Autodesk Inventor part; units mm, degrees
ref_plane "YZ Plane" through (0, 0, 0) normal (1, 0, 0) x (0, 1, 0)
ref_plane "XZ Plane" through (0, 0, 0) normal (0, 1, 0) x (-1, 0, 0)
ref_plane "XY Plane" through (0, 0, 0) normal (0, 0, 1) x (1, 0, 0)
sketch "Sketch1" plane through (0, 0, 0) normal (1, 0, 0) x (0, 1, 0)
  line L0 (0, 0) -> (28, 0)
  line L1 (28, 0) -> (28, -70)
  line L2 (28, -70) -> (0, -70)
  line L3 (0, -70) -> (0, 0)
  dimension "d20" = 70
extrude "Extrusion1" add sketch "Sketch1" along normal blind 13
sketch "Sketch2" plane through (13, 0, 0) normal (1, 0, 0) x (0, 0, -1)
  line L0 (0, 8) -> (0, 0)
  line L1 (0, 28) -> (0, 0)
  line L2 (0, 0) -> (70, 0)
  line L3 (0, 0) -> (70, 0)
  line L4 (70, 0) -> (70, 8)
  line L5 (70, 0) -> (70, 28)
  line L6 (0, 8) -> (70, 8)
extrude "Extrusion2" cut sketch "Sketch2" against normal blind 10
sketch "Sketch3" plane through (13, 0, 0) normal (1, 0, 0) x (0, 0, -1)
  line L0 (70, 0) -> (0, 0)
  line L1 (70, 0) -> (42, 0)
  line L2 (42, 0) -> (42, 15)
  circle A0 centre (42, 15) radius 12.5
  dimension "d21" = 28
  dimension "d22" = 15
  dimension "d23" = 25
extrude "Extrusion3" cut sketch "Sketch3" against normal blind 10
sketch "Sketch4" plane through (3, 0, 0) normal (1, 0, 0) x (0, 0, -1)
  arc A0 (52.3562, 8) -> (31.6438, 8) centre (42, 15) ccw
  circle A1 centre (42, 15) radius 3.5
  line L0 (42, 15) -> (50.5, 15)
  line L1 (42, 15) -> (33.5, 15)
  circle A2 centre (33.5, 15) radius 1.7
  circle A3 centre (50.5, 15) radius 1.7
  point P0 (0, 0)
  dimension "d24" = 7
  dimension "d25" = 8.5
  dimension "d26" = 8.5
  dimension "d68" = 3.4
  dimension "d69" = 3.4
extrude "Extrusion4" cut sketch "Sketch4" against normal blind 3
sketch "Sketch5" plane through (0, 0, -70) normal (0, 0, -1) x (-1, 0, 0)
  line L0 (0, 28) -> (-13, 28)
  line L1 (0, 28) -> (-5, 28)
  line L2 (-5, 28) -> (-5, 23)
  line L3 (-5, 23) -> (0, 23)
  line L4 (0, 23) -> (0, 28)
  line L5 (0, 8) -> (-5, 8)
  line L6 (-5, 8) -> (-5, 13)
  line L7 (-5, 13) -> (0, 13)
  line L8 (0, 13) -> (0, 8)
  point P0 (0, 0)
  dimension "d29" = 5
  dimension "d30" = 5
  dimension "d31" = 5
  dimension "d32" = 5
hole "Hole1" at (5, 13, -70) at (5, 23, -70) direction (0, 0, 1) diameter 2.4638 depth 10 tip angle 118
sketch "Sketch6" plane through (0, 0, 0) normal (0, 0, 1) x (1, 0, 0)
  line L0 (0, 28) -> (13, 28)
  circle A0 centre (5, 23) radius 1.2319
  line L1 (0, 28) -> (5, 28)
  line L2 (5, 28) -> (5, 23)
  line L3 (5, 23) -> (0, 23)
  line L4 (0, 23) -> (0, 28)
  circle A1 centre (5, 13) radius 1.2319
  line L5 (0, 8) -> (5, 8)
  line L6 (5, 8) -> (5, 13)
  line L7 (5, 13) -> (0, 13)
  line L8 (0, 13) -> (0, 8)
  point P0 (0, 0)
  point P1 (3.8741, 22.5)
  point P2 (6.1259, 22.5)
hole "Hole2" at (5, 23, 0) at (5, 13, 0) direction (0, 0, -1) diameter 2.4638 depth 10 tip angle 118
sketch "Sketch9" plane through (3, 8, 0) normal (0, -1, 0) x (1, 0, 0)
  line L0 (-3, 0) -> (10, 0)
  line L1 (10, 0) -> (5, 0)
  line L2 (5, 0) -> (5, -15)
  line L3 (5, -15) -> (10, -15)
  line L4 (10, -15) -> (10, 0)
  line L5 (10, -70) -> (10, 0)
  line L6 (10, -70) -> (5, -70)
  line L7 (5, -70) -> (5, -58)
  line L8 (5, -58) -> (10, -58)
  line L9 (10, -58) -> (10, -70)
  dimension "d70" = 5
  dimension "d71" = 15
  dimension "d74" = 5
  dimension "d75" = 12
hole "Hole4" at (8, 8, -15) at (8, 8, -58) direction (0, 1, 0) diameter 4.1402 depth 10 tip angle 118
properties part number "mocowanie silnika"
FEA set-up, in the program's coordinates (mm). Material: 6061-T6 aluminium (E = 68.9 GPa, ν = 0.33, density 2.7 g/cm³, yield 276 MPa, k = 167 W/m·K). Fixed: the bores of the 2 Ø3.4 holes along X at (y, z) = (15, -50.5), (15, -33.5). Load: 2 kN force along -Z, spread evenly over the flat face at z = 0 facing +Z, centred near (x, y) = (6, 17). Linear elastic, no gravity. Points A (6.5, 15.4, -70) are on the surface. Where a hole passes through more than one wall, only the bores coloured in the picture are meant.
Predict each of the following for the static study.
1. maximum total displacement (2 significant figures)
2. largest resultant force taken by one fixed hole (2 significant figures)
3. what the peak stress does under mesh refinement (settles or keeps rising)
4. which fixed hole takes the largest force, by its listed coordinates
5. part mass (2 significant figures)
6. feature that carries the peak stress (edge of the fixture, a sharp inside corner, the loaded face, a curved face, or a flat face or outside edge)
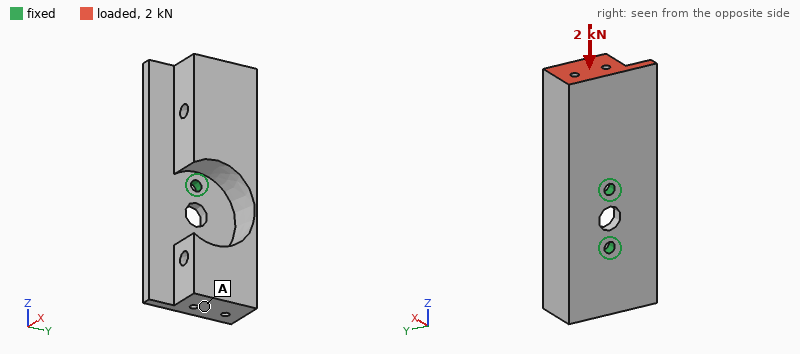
0.17 mm
1.4 kN
keeps rising
(15, -33.5)
41 g
edge of the fixture
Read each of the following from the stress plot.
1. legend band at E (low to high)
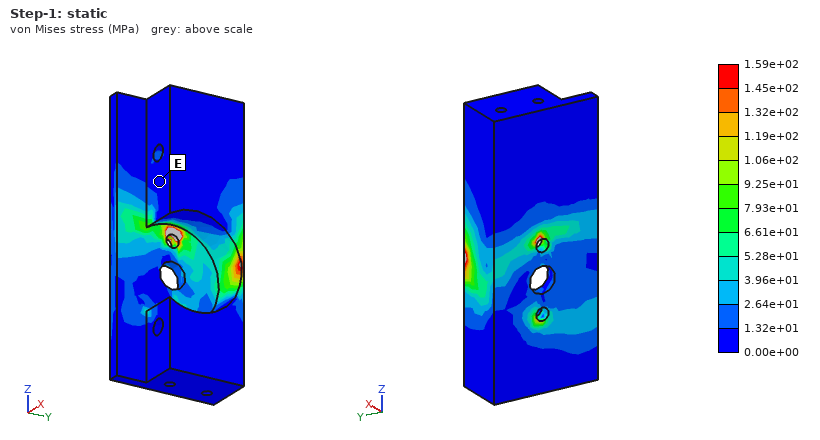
0.00e+00 to 1.32e+01 MPa
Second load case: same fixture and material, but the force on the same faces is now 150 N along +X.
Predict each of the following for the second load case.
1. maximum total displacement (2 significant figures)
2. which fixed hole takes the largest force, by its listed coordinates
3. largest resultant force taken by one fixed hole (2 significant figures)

98 µm
(15, -33.5)
320 N
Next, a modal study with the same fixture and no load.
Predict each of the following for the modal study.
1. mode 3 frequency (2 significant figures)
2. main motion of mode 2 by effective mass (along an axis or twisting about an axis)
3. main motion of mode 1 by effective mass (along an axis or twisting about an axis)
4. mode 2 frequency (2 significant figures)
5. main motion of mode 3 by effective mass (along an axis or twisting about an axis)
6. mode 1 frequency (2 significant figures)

5000 Hz
along Y
along X
4300 Hz
along X
2200 Hz
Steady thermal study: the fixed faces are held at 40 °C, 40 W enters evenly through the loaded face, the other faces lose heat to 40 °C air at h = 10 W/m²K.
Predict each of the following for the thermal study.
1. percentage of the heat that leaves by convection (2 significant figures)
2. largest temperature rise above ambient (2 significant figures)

3.1 %
48 K
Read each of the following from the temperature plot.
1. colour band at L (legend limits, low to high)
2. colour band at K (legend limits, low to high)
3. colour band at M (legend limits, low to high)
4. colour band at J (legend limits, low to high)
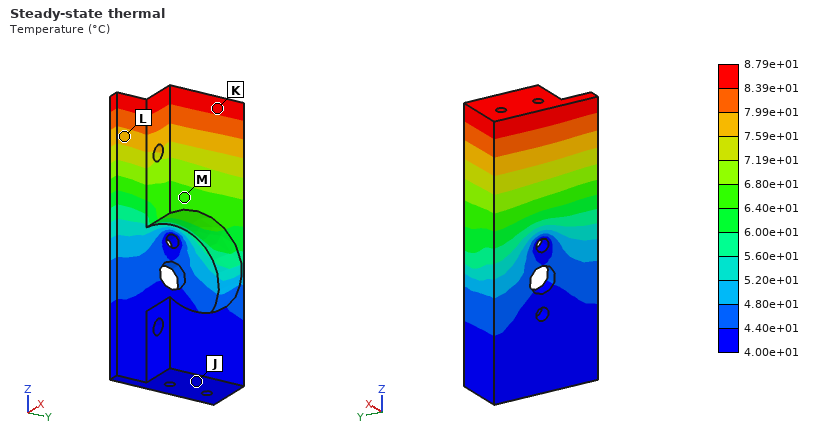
7.59e+01 to 7.99e+01 °C
8.39e+01 to 8.79e+01 °C
6.40e+01 to 6.80e+01 °C
4.00e+01 to 4.40e+01 °C
